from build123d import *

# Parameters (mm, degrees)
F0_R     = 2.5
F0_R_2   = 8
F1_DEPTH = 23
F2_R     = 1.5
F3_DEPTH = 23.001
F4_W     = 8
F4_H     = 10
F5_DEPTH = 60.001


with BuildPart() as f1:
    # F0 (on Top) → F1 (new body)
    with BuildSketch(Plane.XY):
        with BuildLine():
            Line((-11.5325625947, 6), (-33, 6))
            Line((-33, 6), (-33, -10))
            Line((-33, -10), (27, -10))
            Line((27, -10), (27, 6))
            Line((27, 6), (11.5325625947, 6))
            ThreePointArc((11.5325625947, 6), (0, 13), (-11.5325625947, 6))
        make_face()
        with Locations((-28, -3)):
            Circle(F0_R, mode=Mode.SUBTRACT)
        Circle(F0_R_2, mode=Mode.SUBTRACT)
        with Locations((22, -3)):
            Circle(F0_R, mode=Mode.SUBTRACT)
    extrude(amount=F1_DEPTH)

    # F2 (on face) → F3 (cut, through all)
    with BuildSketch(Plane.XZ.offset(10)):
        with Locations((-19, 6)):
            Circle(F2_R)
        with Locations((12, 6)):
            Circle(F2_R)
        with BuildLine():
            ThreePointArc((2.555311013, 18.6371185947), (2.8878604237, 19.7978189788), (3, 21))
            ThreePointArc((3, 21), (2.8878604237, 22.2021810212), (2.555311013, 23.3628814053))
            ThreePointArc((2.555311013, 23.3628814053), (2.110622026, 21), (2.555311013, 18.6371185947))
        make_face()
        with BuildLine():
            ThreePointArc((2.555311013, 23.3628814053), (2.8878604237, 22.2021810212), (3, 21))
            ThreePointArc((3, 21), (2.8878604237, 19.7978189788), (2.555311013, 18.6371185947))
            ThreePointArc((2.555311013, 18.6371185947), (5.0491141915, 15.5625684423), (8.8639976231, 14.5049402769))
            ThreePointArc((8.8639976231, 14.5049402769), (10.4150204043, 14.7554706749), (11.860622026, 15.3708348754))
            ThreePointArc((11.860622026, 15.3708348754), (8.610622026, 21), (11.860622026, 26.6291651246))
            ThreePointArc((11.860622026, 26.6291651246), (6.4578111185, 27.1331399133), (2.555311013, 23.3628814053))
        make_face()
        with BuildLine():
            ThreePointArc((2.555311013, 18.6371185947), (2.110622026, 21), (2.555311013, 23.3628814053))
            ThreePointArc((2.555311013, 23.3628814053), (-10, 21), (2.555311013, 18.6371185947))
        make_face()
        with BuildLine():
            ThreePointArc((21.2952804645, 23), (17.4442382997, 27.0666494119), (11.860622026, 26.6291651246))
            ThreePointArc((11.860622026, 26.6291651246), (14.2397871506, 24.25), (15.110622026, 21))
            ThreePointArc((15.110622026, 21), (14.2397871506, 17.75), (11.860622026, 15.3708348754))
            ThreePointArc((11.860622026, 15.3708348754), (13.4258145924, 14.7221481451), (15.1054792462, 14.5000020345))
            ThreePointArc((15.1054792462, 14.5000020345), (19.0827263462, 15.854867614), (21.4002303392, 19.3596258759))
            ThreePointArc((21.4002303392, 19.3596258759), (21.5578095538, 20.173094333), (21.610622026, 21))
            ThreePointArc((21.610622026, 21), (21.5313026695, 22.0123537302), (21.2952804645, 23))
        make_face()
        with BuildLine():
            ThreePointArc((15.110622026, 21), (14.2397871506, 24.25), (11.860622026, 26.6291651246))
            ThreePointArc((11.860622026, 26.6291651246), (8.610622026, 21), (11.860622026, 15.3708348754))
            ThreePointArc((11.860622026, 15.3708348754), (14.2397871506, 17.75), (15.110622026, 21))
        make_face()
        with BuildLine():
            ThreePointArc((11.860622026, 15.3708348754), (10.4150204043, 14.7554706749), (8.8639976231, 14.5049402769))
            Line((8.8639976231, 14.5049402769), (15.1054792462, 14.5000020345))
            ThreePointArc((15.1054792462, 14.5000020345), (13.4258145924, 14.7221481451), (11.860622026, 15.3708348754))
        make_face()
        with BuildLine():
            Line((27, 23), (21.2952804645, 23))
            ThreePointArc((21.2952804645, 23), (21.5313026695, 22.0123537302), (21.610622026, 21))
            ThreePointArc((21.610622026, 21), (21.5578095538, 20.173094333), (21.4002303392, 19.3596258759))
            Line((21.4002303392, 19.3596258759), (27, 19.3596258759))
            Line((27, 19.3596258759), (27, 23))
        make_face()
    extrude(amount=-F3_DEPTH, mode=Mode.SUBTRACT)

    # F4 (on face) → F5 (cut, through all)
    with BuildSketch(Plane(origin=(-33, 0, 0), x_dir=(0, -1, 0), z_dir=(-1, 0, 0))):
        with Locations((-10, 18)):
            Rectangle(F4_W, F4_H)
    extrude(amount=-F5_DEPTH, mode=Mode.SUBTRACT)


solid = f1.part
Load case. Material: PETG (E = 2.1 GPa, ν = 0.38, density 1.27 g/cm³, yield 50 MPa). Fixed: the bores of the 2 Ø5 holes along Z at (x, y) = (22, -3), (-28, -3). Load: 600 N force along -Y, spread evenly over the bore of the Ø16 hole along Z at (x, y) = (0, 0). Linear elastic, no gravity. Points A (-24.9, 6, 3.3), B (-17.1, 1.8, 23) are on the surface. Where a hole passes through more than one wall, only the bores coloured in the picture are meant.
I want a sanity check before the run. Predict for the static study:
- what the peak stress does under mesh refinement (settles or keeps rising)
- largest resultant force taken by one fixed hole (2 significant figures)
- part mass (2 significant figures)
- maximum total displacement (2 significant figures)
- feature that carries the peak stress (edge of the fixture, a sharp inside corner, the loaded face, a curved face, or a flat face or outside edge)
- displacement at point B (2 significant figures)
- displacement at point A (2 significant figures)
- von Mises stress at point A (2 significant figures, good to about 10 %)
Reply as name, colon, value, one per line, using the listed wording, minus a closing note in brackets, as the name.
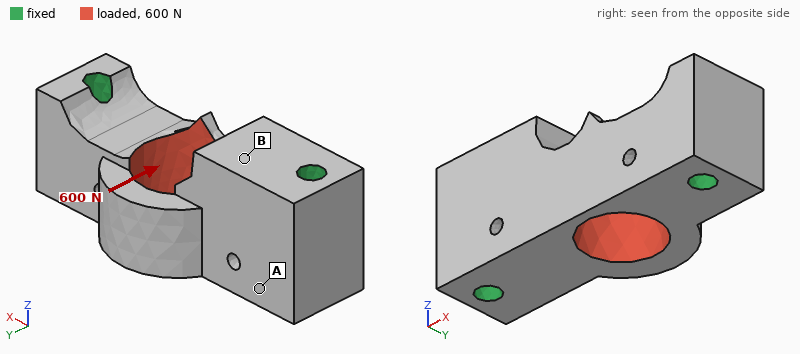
what the peak stress does under mesh refinement: keeps rising
largest resultant force taken by one fixed hole: 310 N
part mass: 19 g
maximum total displacement: 0.11 mm
feature that carries the peak stress: a sharp inside corner
displacement at point B: 0.033 mm
displacement at point A: 0.027 mm
von Mises stress at point A: 2.3 MPa
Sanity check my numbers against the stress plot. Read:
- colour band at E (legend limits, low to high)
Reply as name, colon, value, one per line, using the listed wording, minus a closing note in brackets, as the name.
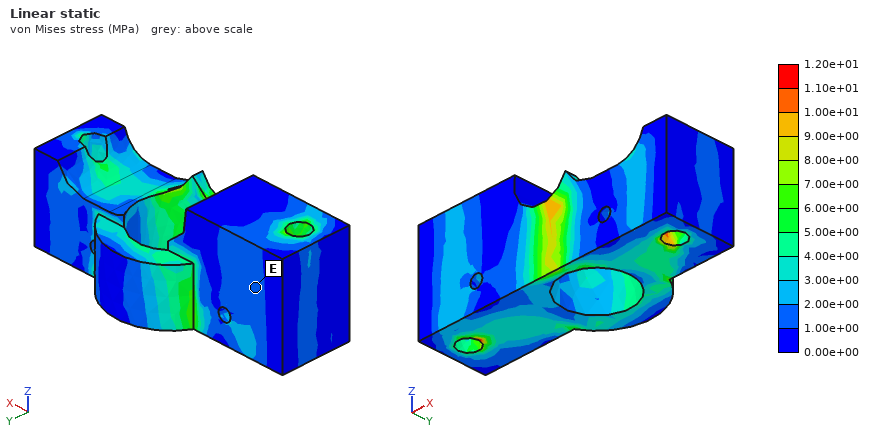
colour band at E: 1.00e+00 to 2.00e+00 MPa
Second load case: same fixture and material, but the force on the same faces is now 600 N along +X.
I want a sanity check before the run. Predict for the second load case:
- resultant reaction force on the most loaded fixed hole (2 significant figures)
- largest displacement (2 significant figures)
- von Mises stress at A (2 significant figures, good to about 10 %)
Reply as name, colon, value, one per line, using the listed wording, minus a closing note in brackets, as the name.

resultant reaction force on the most loaded fixed hole: 300 N
largest displacement: 26 µm
von Mises stress at A: 0.51 MPa
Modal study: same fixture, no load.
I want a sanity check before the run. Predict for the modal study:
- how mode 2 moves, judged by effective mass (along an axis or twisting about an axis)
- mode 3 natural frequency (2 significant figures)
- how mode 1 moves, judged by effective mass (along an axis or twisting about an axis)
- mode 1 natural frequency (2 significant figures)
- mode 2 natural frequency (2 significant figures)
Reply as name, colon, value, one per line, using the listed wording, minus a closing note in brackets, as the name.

how mode 2 moves, judged by effective mass: along Z
mode 3 natural frequency: 7100 Hz
how mode 1 moves, judged by effective mass: along Y
mode 1 natural frequency: 4800 Hz
mode 2 natural frequency: 5600 Hz
